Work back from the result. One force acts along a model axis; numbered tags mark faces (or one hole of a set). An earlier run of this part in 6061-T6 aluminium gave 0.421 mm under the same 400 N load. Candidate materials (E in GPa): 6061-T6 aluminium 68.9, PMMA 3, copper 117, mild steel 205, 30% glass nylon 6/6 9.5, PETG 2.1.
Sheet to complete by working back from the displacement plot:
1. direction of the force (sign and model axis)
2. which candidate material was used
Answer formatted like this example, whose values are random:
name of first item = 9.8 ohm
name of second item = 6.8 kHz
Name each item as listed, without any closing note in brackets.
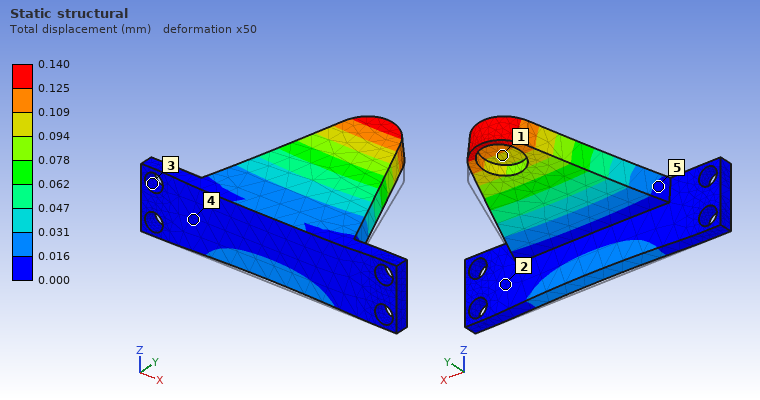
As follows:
direction of the force = +Z
which candidate material was used = mild steel
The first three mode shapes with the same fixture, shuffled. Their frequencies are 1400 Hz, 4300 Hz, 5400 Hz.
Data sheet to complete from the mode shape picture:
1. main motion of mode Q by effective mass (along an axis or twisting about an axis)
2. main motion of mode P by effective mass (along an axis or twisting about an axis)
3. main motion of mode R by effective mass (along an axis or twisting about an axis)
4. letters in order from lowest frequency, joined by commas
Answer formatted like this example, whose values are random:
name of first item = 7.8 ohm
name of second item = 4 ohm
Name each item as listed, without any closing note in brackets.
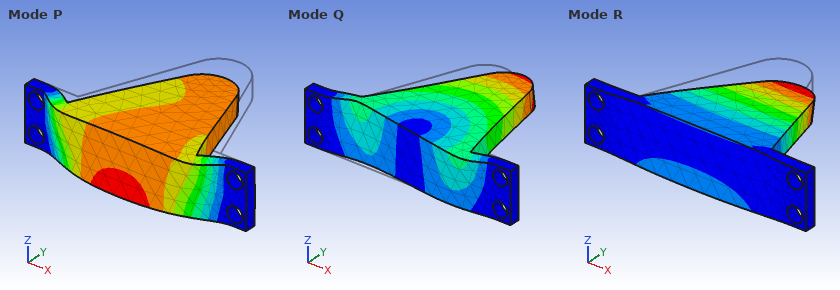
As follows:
main motion of mode Q by effective mass = along X
main motion of mode P by effective mass = along Y
main motion of mode R by effective mass = along Z
letters in order from lowest frequency, joined by commas = R, P, Q
